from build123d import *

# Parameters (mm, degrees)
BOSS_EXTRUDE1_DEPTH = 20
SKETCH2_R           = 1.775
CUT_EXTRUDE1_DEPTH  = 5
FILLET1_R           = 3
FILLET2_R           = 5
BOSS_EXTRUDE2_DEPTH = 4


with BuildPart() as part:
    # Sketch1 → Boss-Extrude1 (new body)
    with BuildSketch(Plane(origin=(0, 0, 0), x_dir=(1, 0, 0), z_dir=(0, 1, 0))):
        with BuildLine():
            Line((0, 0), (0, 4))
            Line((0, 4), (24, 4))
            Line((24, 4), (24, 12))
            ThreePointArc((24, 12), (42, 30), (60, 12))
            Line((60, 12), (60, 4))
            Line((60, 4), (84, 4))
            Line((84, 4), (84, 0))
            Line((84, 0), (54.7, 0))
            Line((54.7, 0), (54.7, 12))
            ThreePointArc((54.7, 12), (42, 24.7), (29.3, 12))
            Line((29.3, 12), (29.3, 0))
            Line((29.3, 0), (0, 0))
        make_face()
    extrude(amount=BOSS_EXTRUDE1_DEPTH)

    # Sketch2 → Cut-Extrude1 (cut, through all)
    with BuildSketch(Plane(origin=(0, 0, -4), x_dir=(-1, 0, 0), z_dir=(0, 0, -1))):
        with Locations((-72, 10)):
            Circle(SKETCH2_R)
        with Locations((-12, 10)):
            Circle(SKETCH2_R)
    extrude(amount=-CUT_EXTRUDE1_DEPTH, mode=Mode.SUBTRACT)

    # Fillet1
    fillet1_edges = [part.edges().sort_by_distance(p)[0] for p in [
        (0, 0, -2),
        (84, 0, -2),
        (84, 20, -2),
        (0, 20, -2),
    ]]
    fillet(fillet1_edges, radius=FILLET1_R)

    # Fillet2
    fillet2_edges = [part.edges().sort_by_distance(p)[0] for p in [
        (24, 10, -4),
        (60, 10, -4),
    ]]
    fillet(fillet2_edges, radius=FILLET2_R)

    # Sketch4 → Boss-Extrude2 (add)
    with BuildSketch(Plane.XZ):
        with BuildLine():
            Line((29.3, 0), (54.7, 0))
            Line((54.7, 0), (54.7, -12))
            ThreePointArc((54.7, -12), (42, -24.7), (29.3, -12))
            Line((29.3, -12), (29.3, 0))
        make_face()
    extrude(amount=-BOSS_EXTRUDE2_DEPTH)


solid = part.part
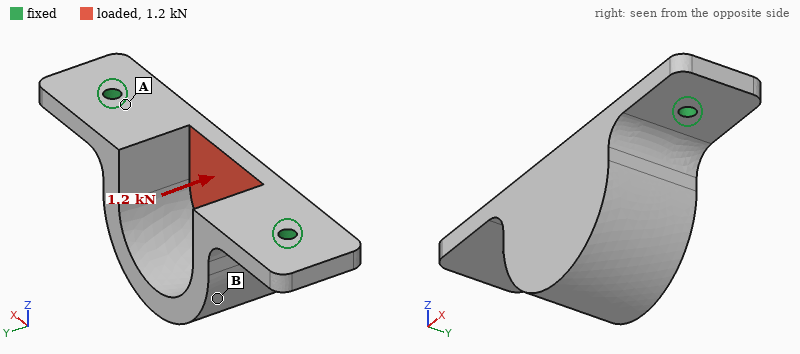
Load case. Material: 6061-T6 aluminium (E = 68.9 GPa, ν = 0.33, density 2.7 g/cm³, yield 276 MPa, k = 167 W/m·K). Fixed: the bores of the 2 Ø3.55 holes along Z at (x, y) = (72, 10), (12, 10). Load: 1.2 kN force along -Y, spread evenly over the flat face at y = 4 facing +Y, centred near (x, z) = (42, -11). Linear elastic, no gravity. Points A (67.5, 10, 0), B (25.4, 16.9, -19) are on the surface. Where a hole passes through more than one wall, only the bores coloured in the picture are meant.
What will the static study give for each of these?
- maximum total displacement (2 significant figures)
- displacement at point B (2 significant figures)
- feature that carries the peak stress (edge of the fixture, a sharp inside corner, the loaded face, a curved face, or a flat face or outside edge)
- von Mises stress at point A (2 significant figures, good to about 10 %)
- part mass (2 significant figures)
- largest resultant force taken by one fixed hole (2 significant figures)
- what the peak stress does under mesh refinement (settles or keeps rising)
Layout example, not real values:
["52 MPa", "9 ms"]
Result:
["0.17 mm", "0.11 mm", "edge of the fixture", "43 MPa", "37 g", "920 N", "keeps rising"]
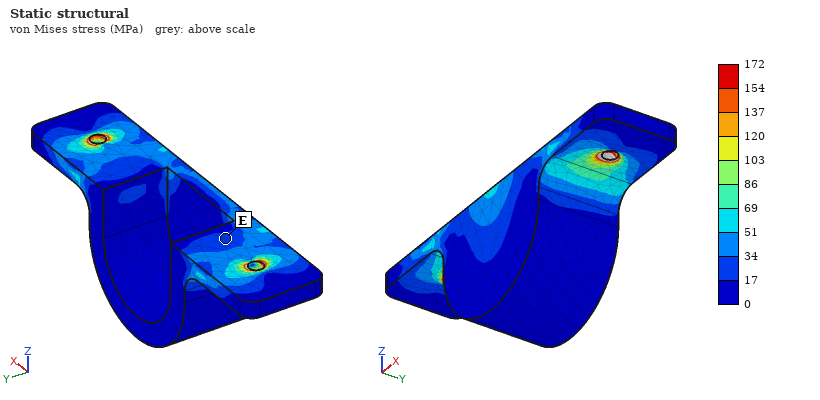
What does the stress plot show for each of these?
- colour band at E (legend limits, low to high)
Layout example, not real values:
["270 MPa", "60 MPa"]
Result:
["17 to 34 MPa"]
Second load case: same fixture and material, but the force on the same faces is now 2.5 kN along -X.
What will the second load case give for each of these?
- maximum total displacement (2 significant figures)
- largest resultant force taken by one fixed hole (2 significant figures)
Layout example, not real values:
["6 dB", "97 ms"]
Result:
["22 µm", "1.3 kN"]
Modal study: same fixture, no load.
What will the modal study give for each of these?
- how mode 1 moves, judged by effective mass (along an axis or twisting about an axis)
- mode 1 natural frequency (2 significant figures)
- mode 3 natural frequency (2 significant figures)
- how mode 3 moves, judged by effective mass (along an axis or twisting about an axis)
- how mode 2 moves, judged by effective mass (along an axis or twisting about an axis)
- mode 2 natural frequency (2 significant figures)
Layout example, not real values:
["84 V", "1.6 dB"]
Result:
["along Y", "2500 Hz", "8600 Hz", "along X", "along Z", "7000 Hz"]
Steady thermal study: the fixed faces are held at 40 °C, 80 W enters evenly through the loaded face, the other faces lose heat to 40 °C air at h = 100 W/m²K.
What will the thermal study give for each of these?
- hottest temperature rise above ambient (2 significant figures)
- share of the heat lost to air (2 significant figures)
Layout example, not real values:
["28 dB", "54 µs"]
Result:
["62 K", "25 %"]
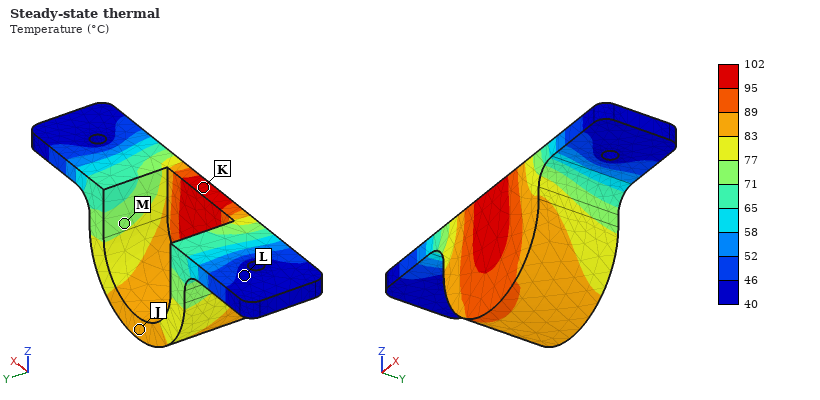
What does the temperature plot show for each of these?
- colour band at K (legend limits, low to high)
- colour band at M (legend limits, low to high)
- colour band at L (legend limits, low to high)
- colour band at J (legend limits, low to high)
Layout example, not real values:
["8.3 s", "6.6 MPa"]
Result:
["95 to 102 °C", "71 to 77 °C", "40 to 46 °C", "83 to 89 °C"]
